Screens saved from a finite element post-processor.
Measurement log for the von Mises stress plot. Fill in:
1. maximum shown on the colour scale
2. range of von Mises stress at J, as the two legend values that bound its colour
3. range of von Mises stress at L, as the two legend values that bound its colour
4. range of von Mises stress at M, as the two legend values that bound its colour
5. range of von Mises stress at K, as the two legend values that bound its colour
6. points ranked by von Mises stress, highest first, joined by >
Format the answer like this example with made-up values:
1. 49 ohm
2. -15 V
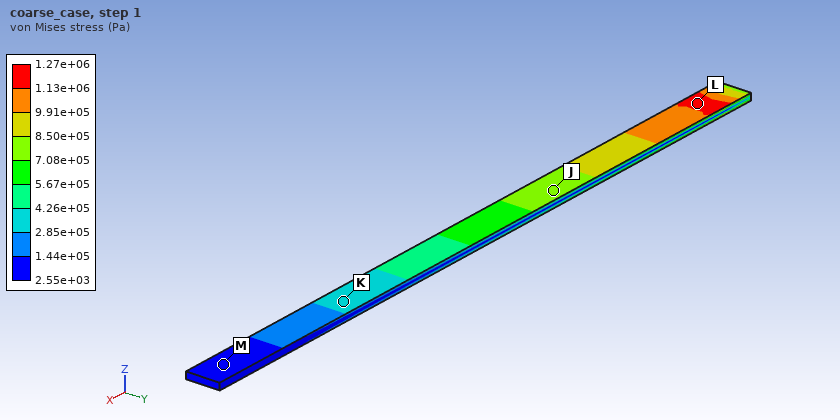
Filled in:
1. 1.27e+06 Pa
2. 7.08e+05 to 8.50e+05 Pa
3. 1.13e+06 to 1.27e+06 Pa
4. 2.55e+03 to 1.44e+05 Pa
5. 2.85e+05 to 4.26e+05 Pa
6. L > J > K > M
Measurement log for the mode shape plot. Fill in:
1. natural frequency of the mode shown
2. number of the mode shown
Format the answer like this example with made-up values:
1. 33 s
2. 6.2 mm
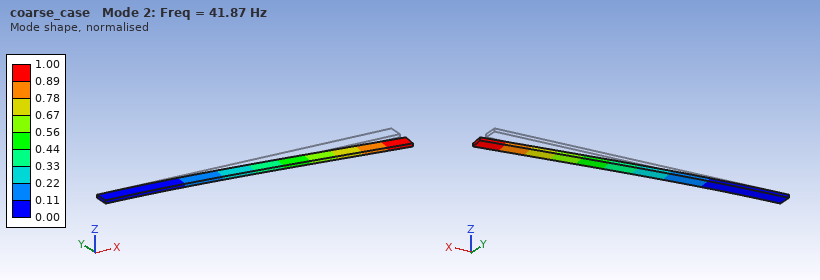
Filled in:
1. 41.87 Hz
2. 2
